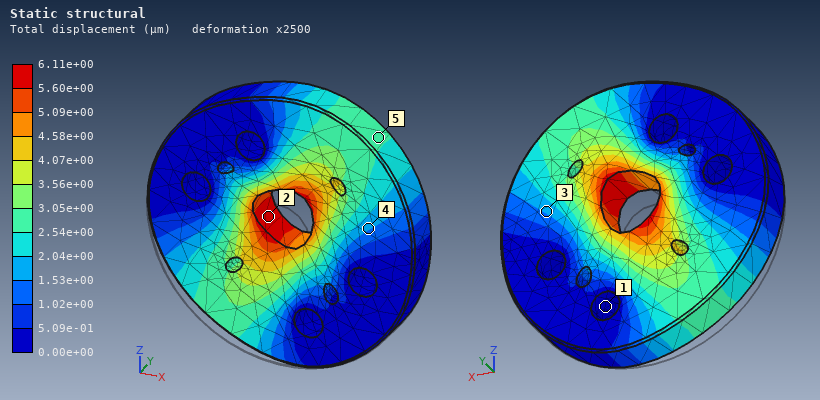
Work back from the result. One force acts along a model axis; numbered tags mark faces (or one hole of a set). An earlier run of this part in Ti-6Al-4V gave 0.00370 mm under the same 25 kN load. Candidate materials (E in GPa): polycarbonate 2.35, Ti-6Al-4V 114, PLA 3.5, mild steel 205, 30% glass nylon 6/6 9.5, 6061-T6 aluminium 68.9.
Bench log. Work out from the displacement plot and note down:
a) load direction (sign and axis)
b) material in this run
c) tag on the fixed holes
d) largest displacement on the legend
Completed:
+Z
6061-T6 aluminium
1
6.11e+00 µm
